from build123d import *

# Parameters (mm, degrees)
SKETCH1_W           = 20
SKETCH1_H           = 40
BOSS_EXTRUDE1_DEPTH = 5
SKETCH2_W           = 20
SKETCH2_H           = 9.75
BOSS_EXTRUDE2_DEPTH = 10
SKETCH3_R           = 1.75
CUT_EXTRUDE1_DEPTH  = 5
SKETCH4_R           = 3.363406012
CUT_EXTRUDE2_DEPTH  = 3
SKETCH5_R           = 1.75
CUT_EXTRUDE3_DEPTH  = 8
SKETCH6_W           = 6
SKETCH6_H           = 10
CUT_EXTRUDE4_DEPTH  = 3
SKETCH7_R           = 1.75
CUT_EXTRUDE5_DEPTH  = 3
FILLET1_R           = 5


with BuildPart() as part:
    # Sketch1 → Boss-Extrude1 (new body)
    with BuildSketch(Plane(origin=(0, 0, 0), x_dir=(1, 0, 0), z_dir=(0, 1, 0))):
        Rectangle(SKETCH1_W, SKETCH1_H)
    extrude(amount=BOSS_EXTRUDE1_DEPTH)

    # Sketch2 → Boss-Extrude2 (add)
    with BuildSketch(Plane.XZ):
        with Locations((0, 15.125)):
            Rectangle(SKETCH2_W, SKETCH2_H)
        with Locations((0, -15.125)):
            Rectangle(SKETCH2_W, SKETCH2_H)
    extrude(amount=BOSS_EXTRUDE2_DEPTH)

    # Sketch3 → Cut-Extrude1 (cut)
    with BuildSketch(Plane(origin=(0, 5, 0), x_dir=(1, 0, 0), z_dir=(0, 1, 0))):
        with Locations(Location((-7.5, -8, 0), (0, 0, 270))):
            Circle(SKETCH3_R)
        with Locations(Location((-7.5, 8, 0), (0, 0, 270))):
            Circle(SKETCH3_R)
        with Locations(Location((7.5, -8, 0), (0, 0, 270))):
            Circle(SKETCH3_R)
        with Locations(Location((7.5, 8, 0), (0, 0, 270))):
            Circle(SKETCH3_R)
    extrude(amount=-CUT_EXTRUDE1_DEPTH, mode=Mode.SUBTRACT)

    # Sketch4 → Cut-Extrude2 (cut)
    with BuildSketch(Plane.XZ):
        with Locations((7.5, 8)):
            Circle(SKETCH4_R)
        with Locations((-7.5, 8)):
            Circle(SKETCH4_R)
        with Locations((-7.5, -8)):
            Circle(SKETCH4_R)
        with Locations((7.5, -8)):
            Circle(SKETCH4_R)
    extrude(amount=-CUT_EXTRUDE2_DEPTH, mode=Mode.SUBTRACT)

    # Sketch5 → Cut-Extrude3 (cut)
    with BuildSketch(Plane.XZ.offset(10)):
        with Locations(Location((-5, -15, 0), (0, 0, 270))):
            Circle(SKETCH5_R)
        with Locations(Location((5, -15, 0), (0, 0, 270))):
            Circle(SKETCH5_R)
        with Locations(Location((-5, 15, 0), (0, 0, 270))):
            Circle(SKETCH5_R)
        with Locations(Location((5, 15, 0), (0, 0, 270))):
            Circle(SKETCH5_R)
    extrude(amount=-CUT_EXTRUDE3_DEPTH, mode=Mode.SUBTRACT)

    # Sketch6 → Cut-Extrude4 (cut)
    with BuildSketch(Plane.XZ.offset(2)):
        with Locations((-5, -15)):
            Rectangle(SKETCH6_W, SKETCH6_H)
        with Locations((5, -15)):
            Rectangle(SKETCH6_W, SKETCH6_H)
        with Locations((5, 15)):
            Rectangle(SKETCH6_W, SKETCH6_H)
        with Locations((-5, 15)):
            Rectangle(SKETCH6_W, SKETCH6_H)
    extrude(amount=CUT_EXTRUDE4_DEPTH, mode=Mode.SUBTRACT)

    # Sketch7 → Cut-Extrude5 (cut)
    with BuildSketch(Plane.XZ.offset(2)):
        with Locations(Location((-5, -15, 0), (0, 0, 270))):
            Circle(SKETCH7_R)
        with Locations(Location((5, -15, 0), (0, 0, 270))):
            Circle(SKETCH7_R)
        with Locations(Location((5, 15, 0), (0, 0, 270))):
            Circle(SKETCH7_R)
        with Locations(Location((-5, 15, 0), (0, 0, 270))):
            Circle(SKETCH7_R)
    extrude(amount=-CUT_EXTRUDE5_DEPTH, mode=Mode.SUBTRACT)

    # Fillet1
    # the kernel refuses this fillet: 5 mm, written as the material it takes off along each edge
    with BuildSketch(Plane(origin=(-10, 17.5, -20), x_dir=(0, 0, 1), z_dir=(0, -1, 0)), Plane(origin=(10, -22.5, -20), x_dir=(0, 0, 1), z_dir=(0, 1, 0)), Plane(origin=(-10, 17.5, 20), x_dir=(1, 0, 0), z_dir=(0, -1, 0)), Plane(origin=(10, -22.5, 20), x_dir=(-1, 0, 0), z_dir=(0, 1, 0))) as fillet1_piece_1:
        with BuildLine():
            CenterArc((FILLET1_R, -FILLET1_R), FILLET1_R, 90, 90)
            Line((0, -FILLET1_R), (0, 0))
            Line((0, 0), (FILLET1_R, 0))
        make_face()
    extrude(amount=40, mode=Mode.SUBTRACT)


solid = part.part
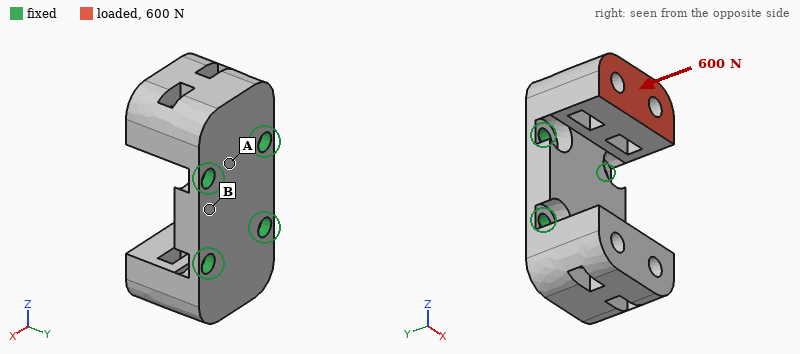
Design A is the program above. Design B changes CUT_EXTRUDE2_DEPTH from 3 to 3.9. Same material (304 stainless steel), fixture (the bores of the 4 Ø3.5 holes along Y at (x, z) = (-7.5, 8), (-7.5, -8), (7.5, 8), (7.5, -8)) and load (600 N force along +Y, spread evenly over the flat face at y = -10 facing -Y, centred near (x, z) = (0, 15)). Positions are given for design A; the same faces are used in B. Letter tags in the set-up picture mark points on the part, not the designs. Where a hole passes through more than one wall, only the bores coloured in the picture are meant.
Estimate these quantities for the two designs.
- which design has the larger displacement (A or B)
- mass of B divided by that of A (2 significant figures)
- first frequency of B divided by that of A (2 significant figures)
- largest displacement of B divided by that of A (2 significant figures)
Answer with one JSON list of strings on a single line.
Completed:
["B", "0.99", "0.86", "1.3"]
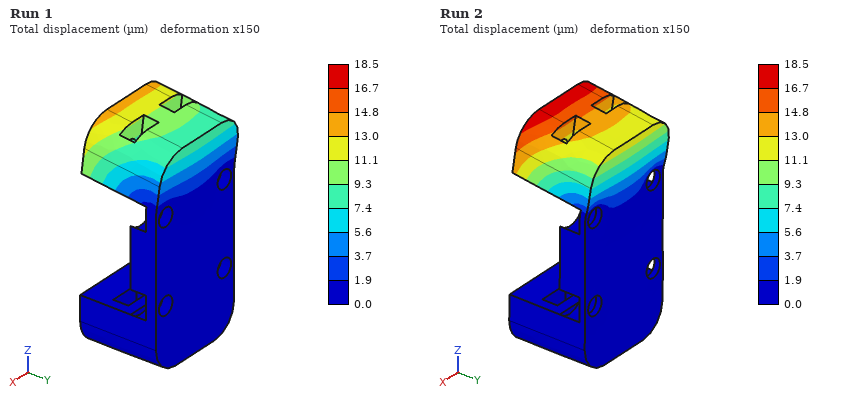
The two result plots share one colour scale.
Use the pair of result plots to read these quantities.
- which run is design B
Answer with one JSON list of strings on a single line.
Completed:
["Run 2"]
